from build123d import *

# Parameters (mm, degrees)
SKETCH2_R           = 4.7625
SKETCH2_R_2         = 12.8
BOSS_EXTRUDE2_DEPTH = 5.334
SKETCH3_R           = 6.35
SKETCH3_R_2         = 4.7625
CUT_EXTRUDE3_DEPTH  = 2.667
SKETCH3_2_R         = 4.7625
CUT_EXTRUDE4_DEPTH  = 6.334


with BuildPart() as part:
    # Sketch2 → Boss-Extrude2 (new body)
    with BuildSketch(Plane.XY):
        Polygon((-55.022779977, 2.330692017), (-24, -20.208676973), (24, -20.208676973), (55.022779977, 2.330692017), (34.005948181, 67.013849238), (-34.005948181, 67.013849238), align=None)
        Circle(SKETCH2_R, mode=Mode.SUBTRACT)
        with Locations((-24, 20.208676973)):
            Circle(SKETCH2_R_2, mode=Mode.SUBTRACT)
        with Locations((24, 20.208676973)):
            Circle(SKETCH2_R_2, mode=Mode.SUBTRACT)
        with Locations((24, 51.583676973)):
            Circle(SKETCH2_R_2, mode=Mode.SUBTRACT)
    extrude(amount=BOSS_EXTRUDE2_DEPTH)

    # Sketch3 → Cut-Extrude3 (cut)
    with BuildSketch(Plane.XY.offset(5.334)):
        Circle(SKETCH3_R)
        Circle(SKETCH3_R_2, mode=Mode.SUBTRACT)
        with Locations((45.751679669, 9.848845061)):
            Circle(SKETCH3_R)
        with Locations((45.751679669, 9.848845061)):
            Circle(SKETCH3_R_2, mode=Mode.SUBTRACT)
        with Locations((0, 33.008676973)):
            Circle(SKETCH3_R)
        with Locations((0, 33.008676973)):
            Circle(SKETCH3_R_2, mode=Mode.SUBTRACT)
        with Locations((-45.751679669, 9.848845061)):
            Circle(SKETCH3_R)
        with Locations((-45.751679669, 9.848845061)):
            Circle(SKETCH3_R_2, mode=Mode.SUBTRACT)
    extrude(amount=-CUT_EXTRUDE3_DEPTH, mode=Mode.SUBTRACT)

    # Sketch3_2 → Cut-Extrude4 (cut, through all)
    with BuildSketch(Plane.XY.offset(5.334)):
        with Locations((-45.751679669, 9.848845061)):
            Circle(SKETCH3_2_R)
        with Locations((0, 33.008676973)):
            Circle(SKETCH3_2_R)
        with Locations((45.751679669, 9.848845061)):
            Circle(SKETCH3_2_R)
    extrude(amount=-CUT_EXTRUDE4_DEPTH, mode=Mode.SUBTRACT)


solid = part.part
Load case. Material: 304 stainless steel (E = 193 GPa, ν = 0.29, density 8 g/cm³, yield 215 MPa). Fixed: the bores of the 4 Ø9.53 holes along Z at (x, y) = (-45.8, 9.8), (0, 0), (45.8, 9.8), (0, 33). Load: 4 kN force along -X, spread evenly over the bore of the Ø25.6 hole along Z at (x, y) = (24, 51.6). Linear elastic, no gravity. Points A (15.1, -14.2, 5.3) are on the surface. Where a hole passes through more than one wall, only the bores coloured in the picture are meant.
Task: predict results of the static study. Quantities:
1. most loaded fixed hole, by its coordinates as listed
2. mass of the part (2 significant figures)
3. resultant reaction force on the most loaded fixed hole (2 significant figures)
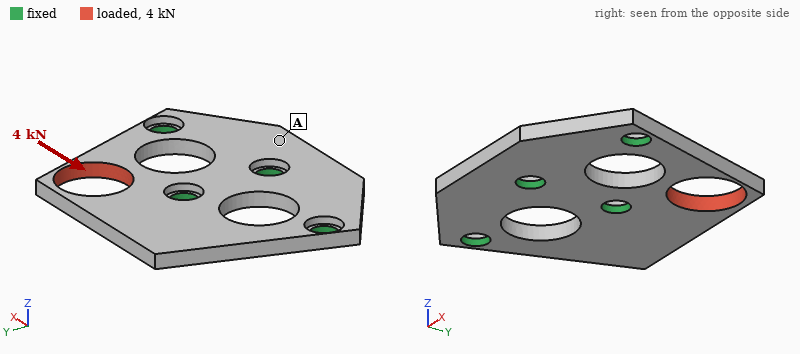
(0, 33)
240 g
3.5 kN
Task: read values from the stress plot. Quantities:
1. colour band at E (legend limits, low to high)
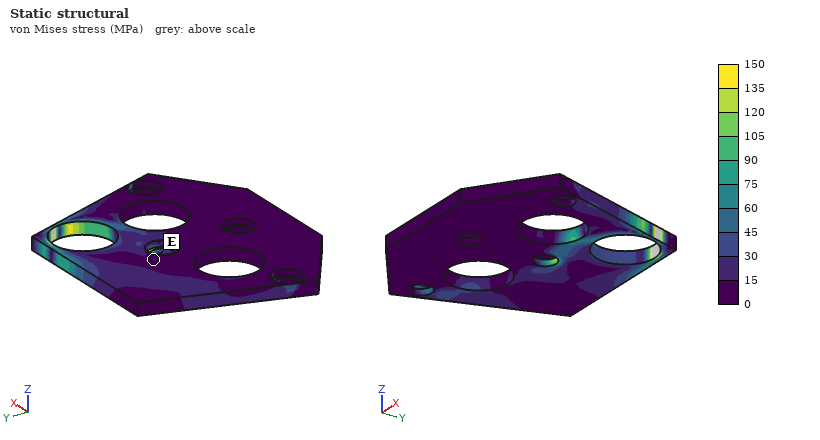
0 to 15 MPa
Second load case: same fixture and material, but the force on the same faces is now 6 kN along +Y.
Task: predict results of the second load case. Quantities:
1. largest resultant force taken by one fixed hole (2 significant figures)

3.0 kN
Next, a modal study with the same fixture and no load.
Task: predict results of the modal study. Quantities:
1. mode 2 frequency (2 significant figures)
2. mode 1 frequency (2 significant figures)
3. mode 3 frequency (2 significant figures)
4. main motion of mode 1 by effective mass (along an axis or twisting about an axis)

3300 Hz
2300 Hz
5600 Hz
along Z
